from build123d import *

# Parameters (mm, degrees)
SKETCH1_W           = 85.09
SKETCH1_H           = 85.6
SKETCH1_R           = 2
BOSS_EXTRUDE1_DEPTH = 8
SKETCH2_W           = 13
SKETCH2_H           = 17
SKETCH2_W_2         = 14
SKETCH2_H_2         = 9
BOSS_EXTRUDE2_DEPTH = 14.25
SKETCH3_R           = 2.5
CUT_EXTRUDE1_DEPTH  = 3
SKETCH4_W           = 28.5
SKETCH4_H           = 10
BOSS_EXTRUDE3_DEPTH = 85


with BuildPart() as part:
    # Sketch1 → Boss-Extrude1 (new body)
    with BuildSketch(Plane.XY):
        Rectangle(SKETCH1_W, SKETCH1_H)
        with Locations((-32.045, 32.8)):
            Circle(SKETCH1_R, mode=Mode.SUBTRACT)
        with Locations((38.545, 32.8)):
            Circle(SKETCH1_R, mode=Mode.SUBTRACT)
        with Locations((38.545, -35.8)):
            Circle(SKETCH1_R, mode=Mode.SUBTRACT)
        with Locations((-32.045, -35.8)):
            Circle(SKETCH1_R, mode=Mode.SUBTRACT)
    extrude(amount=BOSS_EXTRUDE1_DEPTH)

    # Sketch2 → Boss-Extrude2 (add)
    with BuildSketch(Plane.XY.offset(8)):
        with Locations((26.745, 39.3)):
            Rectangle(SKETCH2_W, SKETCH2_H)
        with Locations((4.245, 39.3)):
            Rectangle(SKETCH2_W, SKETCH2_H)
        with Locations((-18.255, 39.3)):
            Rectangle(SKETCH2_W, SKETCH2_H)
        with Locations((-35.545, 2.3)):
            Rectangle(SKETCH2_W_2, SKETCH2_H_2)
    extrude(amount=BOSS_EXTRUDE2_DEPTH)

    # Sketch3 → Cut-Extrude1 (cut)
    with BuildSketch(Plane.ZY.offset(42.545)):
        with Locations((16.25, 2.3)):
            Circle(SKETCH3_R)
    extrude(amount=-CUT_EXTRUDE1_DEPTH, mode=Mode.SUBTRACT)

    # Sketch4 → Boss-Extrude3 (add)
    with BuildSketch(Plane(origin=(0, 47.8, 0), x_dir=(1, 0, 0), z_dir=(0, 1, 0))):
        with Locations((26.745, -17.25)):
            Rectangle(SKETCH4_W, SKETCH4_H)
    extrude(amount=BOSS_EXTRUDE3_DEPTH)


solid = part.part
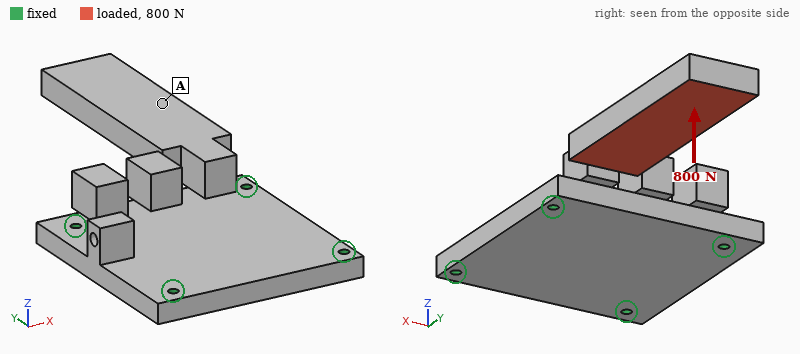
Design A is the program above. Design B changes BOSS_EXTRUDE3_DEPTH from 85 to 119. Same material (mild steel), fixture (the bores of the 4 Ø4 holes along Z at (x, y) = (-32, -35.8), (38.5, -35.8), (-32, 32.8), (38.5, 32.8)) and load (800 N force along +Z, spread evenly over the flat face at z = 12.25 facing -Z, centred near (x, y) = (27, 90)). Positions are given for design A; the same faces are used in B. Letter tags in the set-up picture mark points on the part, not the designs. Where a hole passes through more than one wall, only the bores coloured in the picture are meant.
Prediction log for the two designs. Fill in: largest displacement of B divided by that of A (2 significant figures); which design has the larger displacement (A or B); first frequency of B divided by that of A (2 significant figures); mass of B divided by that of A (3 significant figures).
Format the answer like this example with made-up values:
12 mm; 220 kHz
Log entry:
2.1; B; 0.59; 1.10
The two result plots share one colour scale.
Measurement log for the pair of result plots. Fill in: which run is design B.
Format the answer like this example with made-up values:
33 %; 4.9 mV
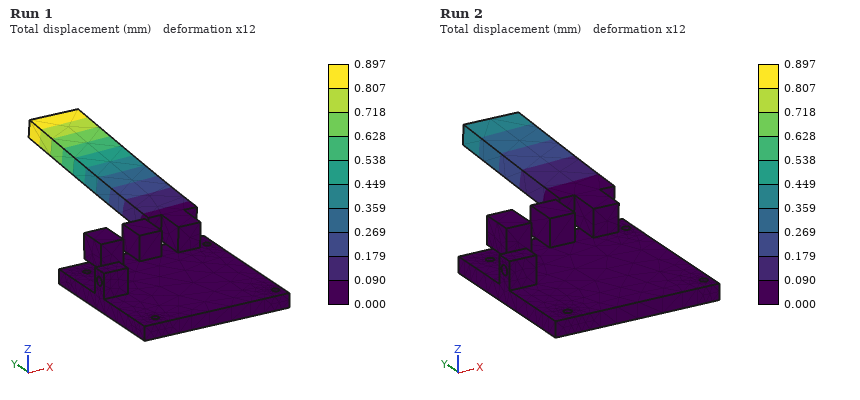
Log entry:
Run 1
